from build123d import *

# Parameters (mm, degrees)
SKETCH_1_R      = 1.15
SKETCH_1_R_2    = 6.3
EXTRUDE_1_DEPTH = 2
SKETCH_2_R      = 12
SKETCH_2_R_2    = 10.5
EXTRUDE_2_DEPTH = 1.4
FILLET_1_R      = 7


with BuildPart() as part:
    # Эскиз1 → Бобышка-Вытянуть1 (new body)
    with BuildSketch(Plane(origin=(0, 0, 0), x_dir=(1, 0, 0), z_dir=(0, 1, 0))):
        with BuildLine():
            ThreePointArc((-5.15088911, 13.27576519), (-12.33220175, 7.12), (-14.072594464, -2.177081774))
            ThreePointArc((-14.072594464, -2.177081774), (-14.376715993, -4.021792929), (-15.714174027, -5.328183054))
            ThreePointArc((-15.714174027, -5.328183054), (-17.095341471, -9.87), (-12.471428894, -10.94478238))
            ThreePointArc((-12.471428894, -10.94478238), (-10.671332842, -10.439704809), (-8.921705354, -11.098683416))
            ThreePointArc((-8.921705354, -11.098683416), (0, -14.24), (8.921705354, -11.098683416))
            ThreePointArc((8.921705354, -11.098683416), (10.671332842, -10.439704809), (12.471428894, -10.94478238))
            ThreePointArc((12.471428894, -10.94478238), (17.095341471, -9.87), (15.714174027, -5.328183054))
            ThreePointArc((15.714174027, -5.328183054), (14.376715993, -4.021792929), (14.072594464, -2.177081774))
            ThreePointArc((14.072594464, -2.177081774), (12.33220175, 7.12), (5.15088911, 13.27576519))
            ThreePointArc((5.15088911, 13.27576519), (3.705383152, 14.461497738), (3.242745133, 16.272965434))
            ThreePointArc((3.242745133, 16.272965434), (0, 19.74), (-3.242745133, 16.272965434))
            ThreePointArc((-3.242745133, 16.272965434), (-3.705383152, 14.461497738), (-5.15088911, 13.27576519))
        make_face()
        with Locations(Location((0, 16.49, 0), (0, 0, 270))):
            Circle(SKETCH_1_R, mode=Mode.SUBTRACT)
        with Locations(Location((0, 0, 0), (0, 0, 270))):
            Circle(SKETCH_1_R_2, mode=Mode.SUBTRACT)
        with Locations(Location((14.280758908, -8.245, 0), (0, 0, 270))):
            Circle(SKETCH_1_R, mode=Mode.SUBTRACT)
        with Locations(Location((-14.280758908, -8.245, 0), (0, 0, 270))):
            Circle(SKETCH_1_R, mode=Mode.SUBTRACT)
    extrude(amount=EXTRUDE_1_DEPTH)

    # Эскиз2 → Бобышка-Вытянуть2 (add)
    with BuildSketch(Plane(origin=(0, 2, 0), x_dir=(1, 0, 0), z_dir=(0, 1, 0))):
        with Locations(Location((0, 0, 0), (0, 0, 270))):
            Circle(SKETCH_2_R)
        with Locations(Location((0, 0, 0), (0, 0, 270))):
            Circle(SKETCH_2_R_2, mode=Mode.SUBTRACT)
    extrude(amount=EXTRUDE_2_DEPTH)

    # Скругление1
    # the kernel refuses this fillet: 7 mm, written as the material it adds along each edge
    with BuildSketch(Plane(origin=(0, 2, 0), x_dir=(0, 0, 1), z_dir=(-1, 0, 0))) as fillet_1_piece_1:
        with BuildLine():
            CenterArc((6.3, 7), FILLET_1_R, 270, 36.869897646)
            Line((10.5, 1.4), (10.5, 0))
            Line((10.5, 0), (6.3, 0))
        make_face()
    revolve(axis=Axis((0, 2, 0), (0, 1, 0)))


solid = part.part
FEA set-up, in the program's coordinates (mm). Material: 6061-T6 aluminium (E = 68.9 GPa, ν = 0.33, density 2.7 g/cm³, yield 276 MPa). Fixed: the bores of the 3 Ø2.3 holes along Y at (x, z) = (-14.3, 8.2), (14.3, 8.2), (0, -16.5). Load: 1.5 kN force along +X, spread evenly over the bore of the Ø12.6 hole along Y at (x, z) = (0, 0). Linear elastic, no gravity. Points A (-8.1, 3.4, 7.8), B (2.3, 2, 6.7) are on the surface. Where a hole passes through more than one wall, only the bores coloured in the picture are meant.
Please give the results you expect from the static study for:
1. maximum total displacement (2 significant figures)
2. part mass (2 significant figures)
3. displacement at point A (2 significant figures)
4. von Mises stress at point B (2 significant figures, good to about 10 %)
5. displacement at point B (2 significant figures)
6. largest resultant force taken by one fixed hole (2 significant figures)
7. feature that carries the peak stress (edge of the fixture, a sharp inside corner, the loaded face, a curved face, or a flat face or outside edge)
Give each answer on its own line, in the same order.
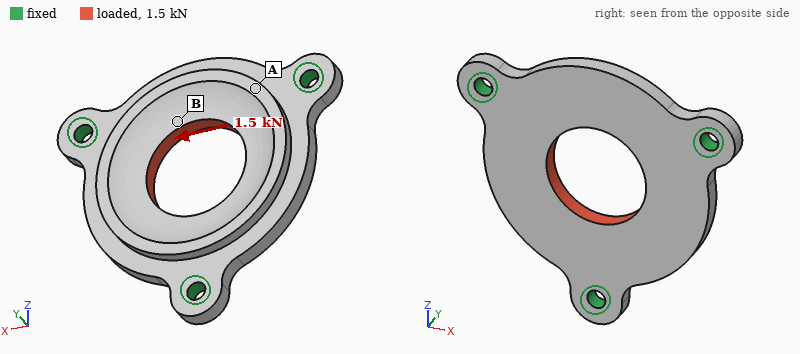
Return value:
15 µm
3.9 g
4.9 µm
42 MPa
4.8 µm
530 N
edge of the fixture
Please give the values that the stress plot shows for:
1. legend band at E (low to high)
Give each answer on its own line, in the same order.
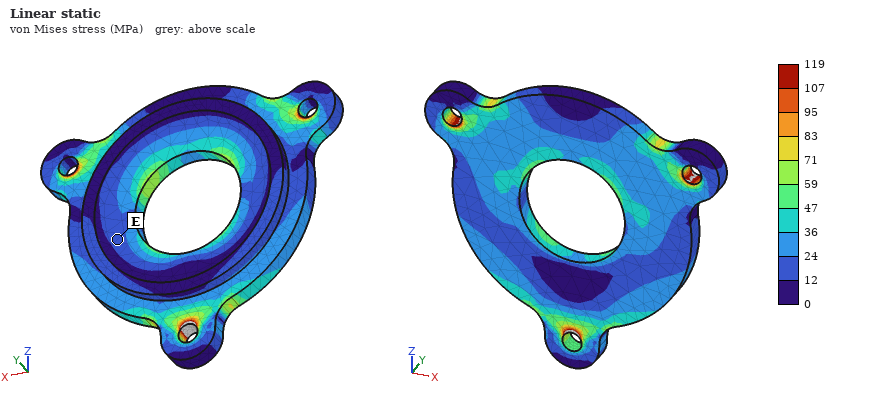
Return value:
12 to 24 MPa
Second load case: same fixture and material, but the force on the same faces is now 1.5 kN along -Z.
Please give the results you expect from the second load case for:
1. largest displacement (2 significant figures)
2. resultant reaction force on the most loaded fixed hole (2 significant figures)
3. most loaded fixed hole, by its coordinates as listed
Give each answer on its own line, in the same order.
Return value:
16 µm
550 N
(0, -16.5)
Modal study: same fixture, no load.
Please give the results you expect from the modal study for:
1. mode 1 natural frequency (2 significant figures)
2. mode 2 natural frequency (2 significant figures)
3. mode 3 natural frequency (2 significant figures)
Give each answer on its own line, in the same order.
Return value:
13 kHz
13 kHz
13 kHz
